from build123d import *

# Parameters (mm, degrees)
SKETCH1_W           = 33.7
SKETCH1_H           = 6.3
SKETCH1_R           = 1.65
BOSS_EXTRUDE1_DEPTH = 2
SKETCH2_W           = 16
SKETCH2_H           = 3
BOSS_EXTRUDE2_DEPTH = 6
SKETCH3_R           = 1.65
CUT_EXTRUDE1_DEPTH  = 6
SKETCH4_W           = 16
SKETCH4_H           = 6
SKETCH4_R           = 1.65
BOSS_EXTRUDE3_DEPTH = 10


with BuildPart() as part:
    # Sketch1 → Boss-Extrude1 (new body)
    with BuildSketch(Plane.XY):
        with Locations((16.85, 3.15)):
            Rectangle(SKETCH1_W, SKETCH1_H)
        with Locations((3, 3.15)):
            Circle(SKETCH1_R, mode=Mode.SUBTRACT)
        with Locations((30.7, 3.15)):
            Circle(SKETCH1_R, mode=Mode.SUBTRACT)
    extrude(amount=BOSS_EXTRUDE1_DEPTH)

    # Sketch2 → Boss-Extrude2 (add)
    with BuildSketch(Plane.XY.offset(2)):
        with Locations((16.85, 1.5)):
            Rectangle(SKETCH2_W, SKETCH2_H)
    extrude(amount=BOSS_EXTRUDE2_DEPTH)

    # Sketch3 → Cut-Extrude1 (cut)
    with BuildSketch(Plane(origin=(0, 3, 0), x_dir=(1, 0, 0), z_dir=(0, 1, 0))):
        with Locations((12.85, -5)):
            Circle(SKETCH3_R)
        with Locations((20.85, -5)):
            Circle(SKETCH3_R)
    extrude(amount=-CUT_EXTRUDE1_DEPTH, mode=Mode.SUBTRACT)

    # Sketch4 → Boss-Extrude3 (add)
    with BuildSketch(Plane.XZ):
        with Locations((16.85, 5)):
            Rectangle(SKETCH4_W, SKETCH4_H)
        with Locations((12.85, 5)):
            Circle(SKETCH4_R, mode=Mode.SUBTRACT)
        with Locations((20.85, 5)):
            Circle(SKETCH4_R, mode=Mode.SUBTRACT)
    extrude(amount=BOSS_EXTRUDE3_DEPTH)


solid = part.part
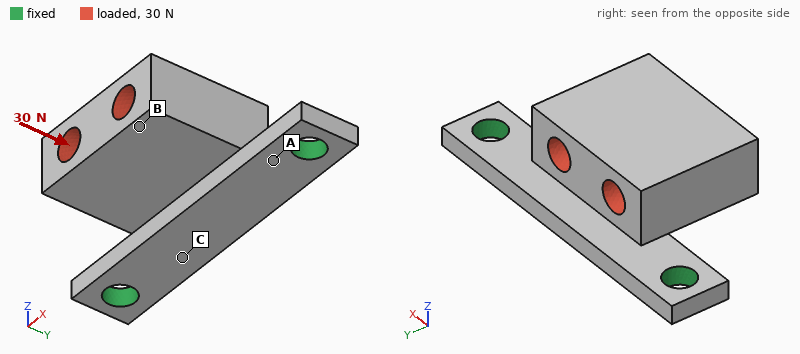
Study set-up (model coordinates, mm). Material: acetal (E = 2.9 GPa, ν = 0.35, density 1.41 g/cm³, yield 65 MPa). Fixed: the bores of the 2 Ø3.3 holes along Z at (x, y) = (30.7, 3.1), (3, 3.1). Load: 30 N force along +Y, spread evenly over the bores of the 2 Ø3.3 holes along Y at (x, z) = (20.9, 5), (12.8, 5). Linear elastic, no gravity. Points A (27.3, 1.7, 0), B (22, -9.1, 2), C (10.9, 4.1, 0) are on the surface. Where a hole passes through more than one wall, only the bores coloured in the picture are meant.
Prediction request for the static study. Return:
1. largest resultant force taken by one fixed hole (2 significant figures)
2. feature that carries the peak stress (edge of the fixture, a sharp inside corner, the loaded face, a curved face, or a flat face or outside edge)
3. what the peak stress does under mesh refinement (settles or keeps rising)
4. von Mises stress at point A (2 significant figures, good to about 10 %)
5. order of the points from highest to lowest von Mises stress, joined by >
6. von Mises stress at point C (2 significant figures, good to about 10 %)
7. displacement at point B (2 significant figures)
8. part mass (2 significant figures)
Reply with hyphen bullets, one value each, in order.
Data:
- 15 N
- edge of the fixture
- keeps rising
- 9.9 MPa
- A > C > B
- 6.1 MPa
- 0.28 mm
- 2.0 g
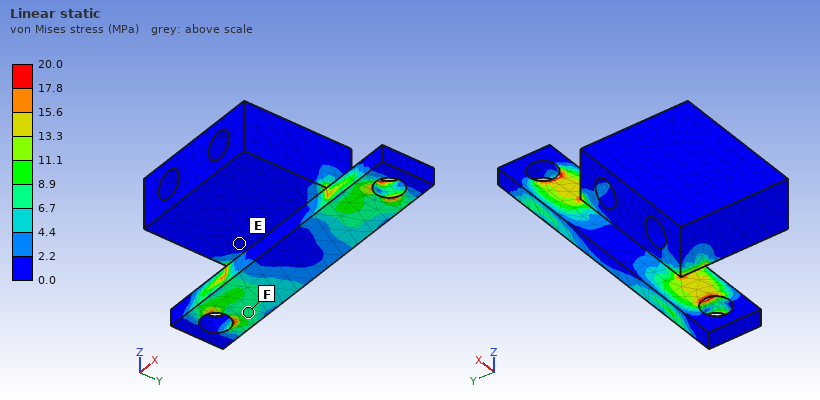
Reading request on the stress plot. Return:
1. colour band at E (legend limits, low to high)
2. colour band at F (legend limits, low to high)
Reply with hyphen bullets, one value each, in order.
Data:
- 0.0 to 2.2 MPa
- 6.7 to 8.9 MPa
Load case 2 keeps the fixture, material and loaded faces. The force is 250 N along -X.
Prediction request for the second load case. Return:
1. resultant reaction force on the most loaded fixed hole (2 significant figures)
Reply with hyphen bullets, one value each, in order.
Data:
- 150 N
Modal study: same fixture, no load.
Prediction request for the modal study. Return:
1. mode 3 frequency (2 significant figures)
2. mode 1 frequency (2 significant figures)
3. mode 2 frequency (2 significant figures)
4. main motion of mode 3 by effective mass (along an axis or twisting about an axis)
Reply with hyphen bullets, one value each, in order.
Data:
- 5000 Hz
- 1100 Hz
- 4300 Hz
- along X
